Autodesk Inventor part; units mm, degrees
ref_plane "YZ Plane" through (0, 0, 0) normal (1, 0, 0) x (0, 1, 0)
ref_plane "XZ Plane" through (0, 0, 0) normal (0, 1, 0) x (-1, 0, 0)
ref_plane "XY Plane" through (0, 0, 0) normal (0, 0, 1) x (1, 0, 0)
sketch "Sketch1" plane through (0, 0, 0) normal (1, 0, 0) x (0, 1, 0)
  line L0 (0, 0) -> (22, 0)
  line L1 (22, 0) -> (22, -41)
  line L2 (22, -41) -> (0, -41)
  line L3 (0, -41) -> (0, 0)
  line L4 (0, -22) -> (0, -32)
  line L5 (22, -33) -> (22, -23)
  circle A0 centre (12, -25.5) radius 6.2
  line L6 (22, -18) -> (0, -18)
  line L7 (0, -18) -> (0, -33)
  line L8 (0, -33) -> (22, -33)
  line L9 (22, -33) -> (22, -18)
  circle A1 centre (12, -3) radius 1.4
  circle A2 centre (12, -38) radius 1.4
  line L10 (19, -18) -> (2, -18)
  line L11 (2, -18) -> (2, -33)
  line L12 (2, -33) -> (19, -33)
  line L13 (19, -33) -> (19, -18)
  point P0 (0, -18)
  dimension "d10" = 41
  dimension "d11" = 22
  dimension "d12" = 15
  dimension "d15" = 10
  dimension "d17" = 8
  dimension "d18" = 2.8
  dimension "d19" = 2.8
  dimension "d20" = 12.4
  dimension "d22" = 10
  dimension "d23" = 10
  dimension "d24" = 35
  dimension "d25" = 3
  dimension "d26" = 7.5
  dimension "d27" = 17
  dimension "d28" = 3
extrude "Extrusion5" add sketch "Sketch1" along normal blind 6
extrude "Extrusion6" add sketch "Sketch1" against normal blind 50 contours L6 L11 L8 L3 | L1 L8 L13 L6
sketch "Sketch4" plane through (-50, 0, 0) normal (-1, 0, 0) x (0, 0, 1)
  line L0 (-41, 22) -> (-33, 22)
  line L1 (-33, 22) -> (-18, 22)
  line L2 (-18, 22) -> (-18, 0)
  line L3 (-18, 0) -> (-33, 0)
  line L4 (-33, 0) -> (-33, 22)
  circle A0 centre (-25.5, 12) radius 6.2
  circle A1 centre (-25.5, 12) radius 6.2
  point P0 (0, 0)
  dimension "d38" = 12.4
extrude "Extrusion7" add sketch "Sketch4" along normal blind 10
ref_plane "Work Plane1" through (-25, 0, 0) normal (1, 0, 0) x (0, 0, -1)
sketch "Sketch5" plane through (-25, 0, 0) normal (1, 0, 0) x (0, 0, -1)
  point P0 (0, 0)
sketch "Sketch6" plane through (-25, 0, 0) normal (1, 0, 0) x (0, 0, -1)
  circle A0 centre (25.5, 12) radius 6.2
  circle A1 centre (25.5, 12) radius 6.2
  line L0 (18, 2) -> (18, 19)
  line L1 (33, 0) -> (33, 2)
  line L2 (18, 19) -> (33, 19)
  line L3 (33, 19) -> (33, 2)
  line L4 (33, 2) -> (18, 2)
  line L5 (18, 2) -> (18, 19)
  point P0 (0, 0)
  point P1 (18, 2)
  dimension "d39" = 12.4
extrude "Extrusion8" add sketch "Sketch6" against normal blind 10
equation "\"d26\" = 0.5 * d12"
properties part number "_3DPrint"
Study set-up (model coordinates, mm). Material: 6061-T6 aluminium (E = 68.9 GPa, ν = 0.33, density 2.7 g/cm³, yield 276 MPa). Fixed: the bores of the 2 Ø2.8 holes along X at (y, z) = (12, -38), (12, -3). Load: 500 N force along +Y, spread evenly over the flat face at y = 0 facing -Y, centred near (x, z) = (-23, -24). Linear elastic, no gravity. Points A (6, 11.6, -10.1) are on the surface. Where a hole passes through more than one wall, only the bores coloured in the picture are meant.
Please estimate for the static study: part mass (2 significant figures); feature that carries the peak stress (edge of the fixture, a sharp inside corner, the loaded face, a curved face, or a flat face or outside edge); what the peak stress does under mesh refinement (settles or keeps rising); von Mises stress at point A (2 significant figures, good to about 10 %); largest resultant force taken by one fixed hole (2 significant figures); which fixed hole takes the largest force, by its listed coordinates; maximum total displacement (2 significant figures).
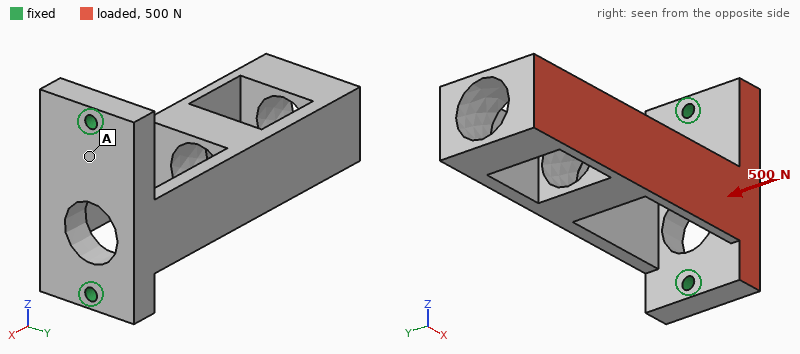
32 g
edge of the fixture
keeps rising
28 MPa
310 N
(12, -38)
0.43 mm
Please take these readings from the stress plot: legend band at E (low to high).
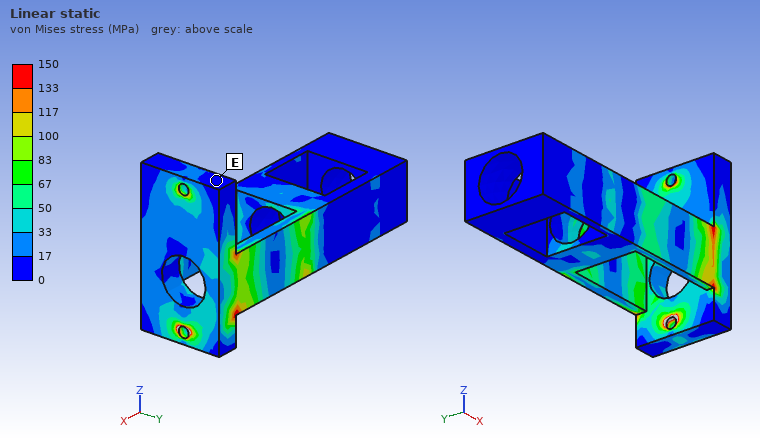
0 to 17 MPa
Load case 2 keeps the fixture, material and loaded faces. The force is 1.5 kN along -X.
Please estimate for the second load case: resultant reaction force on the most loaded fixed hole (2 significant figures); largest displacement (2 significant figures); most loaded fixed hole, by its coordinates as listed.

920 N
0.29 mm
(12, -38)
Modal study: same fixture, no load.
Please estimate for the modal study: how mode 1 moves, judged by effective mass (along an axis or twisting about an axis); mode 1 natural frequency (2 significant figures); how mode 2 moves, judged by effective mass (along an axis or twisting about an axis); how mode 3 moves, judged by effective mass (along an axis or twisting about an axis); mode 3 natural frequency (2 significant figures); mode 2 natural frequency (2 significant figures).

along Y
1200 Hz
along Z
twisting about X
4000 Hz
1700 Hz
